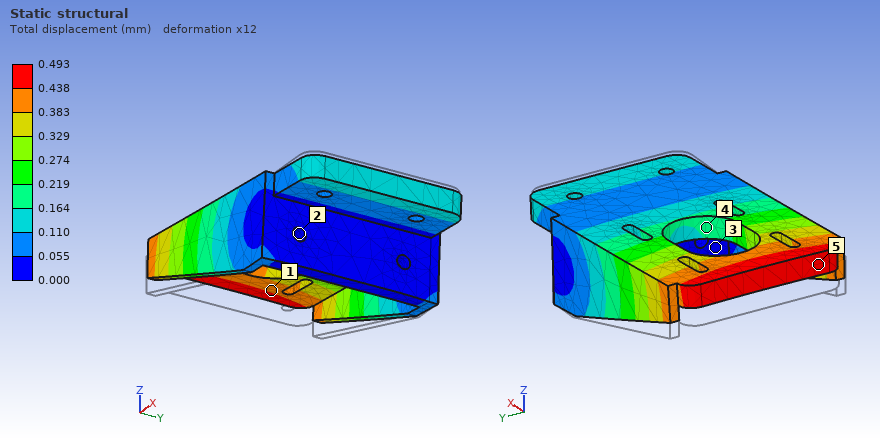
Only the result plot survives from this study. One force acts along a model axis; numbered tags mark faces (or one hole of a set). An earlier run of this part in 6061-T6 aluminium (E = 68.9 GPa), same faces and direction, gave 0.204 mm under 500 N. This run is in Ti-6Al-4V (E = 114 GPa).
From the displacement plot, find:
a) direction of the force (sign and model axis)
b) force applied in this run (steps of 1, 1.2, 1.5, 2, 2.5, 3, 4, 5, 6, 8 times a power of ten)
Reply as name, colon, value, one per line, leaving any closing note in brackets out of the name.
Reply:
direction of the force: +Z
force applied in this run: 2 kN
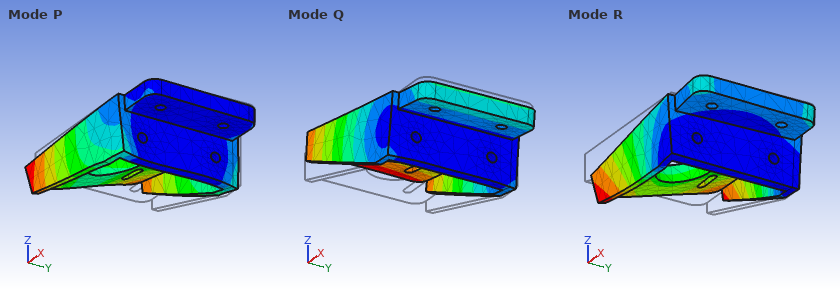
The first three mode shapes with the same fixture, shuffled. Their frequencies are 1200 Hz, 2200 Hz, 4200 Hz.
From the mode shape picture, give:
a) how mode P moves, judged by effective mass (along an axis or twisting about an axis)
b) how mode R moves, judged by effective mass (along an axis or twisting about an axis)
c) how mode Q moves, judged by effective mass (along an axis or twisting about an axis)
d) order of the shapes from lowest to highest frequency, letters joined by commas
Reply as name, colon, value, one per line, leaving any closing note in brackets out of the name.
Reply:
how mode P moves, judged by effective mass: along Y
how mode R moves, judged by effective mass: along Y
how mode Q moves, judged by effective mass: along Z
order of the shapes from lowest to highest frequency, letters joined by commas: Q, R, P
